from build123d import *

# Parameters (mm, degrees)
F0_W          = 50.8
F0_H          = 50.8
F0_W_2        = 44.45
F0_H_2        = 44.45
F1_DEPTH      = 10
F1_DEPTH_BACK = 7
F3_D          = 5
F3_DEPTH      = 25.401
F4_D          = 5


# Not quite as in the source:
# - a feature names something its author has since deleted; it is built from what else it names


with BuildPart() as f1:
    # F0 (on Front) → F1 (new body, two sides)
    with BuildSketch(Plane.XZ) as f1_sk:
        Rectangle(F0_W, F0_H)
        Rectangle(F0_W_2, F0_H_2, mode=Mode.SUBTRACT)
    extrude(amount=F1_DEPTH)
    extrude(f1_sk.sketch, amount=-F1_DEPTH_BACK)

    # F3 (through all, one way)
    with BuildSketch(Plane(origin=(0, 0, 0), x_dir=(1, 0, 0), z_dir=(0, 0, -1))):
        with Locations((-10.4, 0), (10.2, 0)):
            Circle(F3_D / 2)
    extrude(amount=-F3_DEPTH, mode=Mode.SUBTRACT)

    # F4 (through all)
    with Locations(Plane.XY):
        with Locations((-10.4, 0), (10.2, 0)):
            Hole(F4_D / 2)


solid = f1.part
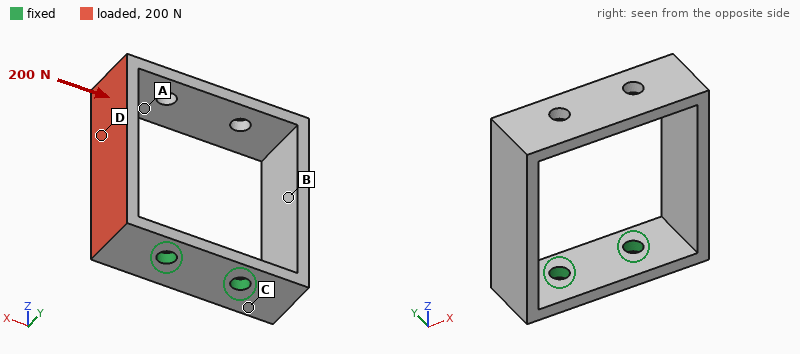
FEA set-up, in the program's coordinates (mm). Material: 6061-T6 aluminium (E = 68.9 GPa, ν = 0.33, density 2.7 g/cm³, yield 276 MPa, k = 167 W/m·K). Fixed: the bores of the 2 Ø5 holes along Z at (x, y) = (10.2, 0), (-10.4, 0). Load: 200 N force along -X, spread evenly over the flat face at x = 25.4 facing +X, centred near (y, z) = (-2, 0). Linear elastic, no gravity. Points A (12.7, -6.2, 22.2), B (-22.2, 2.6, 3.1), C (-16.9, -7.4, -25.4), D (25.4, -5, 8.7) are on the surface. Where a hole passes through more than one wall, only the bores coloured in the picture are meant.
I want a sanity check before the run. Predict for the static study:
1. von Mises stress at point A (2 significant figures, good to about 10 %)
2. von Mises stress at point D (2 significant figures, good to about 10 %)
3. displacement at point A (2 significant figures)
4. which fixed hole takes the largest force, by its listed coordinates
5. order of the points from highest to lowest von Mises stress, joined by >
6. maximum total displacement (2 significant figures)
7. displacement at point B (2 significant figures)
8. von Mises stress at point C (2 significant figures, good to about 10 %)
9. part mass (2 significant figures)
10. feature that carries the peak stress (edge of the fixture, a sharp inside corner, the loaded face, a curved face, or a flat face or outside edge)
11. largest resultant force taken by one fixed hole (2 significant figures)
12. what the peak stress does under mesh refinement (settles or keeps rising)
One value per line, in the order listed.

13 MPa
31 MPa
0.37 mm
(10.2, 0)
C > D > A > B
0.39 mm
0.21 mm
43 MPa
27 g
edge of the fixture
150 N
keeps rising
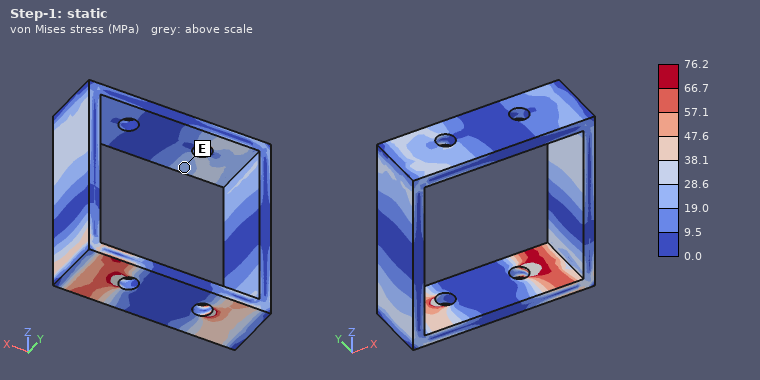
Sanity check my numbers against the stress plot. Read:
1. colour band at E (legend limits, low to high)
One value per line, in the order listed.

19.0 to 28.6 MPa
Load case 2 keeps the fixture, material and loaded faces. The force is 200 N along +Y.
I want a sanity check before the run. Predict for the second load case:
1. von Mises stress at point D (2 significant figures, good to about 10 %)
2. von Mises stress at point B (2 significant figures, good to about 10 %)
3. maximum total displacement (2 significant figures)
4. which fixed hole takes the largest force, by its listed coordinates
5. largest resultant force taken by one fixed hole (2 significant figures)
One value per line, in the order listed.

20 MPa
15 MPa
0.40 mm
(10.2, 0)
270 N
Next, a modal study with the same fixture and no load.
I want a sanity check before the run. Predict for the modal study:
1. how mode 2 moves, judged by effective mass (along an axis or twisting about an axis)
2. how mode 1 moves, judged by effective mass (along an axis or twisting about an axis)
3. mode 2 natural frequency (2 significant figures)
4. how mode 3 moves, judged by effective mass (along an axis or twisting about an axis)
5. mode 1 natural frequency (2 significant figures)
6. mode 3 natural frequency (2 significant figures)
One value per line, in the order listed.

along Y
along X
910 Hz
twisting about Z
760 Hz
1800 Hz
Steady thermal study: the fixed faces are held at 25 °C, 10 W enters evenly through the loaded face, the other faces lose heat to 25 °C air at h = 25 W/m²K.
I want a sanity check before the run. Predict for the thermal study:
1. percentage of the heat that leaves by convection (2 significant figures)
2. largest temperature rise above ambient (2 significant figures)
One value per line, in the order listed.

16 %
23 K
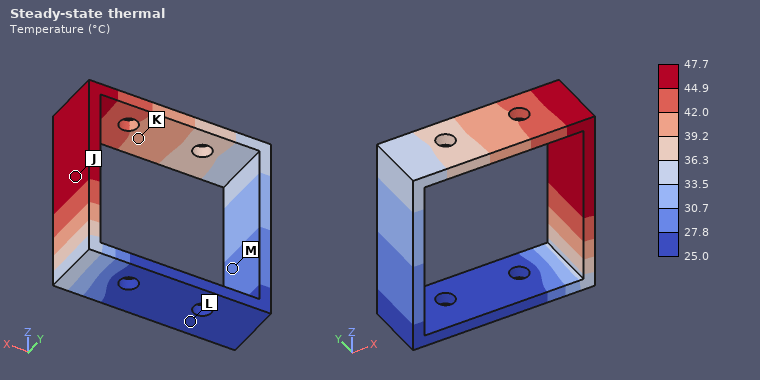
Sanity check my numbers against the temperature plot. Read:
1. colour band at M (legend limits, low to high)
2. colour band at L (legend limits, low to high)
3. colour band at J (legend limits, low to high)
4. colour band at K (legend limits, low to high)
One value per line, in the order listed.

27.8 to 30.7 °C
25.0 to 27.8 °C
44.9 to 47.7 °C
39.2 to 42.0 °C
